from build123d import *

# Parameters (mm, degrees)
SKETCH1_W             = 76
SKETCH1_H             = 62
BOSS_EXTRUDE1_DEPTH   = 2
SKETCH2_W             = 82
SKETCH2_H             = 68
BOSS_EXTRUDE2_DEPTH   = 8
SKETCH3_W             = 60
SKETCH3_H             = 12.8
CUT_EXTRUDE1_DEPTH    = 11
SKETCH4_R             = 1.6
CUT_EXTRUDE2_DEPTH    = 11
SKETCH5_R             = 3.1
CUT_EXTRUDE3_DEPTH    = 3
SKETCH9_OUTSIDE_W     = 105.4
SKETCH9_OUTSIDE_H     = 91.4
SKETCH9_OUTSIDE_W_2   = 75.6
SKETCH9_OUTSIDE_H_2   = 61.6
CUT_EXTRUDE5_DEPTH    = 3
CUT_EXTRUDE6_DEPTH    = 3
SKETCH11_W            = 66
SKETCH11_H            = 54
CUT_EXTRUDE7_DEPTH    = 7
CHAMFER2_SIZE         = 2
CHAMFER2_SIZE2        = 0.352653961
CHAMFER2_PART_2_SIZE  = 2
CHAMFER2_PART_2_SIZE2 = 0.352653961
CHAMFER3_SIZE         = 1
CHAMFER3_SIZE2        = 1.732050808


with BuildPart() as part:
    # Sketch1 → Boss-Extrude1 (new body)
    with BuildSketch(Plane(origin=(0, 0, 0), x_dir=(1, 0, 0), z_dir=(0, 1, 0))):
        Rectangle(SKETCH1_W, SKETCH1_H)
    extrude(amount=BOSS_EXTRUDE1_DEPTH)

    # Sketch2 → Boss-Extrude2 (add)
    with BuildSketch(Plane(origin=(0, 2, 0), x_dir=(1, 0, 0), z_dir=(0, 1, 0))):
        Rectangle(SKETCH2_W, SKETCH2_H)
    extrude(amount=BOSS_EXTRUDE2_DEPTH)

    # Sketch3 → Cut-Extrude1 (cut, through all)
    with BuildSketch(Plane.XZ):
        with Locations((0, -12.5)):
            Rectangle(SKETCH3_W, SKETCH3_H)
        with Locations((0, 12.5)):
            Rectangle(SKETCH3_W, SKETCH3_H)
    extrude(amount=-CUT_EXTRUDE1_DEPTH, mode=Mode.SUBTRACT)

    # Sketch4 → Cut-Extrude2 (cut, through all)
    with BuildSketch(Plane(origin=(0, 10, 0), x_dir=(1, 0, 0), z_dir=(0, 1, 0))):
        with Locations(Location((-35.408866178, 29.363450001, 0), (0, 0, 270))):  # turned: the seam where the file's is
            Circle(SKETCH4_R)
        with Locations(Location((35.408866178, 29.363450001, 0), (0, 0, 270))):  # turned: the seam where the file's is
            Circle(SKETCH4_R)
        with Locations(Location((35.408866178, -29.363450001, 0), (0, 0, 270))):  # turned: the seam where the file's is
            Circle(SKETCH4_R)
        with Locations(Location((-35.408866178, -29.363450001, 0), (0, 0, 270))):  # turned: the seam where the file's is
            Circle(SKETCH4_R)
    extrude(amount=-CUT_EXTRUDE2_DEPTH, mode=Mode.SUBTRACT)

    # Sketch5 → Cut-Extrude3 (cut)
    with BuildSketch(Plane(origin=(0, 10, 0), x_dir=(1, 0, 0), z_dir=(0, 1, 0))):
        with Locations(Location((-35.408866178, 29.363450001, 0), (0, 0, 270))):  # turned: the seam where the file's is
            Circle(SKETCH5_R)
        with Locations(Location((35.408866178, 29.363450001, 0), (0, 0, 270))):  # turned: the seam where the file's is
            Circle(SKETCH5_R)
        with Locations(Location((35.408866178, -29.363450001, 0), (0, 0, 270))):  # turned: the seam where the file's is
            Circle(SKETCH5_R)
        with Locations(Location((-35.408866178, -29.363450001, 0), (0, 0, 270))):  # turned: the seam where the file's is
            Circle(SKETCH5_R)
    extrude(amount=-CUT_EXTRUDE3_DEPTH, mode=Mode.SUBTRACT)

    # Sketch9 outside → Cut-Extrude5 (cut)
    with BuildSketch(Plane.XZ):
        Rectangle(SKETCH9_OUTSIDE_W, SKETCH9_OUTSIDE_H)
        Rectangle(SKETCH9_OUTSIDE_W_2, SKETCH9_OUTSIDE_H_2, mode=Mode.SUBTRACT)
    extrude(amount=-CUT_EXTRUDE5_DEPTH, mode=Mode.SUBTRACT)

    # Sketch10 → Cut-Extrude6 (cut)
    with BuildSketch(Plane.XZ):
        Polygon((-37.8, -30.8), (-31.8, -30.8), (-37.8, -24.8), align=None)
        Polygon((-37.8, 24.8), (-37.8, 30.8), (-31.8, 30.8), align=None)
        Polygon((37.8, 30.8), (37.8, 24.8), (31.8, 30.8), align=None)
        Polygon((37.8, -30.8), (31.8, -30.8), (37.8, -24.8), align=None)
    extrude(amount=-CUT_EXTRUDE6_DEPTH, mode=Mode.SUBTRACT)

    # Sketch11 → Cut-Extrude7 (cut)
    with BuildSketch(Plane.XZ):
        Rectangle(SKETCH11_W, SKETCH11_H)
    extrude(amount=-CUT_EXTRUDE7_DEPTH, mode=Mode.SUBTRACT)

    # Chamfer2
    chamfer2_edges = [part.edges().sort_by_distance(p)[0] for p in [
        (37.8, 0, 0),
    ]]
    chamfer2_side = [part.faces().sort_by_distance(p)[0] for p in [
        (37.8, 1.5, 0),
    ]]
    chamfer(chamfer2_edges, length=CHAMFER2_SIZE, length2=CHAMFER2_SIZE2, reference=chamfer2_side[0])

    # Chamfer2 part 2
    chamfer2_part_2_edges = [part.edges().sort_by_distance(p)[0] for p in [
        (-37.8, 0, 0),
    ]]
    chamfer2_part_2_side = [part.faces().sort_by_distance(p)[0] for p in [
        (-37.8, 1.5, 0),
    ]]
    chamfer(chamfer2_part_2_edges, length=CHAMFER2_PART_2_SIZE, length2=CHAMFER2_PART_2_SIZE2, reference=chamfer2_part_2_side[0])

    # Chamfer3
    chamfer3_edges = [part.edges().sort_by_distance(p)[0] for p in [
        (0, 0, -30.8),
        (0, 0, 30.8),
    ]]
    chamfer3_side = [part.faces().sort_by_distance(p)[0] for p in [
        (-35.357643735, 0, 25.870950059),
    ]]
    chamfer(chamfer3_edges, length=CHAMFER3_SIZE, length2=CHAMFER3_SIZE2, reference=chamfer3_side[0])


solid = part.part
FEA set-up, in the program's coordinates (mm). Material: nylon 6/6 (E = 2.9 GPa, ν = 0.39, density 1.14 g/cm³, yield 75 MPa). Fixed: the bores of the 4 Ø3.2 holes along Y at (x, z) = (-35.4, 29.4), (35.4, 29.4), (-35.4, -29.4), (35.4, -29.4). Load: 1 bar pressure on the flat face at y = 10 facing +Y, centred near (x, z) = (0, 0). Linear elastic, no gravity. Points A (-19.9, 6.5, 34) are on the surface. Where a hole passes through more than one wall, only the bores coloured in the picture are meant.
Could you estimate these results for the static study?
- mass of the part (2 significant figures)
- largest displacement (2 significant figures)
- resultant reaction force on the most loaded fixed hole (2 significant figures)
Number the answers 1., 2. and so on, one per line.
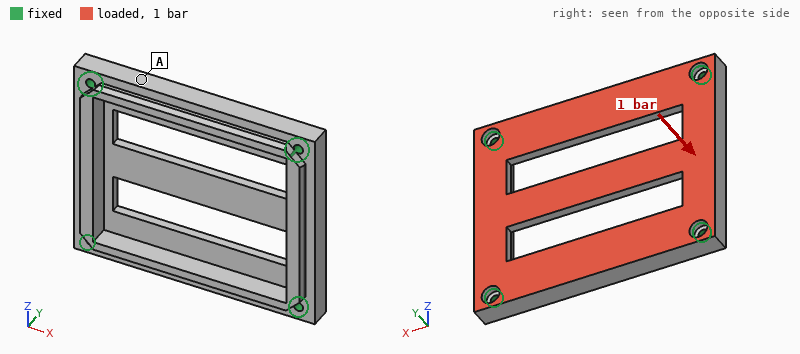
1. 26 g
2. 1.1 mm
3. 110 N
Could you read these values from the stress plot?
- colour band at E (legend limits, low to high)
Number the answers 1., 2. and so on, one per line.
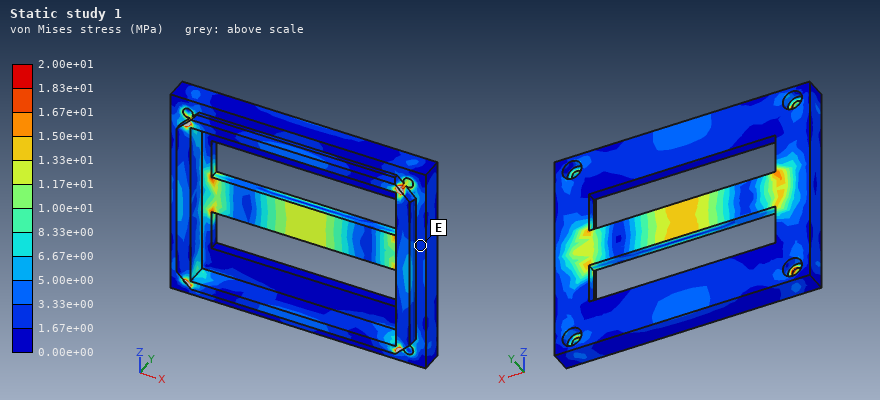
1. 1.67e+00 to 3.33e+00 MPa
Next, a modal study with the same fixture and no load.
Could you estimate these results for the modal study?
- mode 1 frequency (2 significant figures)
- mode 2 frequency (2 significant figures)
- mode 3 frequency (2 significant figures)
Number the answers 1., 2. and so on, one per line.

1. 970 Hz
2. 2100 Hz
3. 2100 Hz
